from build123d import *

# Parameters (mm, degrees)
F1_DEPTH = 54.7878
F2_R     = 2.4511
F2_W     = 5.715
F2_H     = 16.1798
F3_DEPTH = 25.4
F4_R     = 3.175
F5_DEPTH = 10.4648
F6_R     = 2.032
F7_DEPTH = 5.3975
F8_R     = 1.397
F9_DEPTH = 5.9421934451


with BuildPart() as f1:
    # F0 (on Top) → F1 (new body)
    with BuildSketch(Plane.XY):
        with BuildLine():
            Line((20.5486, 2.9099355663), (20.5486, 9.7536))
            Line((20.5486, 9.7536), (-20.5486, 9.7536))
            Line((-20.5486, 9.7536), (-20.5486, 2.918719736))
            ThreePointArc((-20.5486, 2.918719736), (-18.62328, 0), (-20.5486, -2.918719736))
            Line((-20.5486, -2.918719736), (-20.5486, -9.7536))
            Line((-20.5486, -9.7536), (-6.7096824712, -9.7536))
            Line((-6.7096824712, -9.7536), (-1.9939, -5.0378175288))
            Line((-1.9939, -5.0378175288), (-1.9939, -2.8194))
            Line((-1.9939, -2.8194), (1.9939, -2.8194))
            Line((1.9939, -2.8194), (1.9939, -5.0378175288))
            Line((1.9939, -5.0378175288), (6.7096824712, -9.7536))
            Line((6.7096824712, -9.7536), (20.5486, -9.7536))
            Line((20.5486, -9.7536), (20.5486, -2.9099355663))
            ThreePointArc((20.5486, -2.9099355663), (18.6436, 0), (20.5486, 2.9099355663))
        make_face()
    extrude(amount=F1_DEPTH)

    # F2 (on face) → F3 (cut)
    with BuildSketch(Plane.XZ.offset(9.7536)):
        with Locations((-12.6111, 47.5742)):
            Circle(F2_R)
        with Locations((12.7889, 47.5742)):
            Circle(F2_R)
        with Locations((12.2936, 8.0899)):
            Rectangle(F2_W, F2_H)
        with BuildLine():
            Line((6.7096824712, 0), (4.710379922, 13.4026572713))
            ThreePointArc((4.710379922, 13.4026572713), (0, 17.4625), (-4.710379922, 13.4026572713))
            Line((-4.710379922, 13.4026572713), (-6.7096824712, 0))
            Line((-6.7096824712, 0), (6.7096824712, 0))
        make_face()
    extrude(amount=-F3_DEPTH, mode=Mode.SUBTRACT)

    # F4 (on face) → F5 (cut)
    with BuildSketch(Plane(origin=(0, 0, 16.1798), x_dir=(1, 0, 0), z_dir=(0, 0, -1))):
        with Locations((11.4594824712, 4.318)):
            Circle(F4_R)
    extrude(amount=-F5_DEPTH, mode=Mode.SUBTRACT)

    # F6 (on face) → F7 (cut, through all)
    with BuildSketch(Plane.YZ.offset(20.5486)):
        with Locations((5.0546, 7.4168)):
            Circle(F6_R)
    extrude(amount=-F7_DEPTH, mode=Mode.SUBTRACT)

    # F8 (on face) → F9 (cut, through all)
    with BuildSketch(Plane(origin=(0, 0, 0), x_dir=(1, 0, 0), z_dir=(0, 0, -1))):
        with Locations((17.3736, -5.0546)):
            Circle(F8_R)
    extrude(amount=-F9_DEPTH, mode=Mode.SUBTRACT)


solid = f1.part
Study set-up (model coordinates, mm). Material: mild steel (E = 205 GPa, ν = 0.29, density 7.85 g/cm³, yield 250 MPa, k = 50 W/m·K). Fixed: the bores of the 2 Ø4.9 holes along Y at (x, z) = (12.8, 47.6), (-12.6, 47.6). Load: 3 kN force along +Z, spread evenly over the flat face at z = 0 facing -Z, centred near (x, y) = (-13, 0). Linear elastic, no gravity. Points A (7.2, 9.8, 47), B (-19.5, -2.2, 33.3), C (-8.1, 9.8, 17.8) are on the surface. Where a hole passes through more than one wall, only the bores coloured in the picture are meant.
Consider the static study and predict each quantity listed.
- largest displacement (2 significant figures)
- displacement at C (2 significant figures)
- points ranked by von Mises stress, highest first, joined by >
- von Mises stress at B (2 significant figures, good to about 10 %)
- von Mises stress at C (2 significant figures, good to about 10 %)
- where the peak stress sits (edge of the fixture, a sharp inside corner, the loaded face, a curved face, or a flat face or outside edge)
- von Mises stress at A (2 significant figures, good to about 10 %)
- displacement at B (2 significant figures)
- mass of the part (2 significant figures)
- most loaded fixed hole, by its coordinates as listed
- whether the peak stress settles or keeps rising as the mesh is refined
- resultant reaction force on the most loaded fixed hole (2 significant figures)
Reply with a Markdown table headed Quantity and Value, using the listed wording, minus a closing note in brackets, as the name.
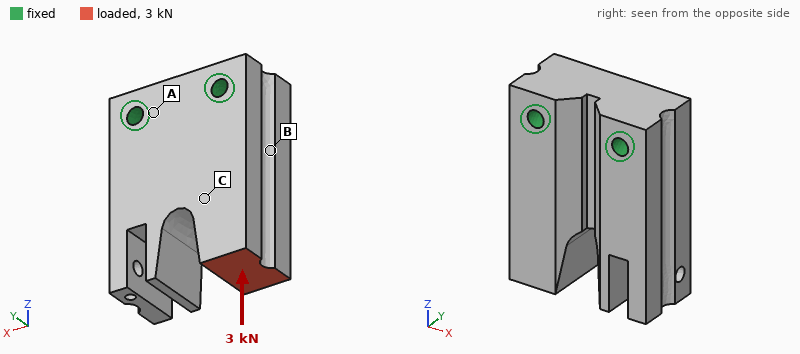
| Quantity | Value |
|---|---|
| largest displacement | 4.4 µm |
| displacement at C | 1.4 µm |
| points ranked by von Mises stress, highest first, joined by > | B > C > A |
| von Mises stress at B | 13 MPa |
| von Mises stress at C | 8.2 MPa |
| where the peak stress sits | edge of the fixture |
| von Mises stress at A | 2.2 MPa |
| displacement at B | 1.0 µm |
| mass of the part | 270 g |
| most loaded fixed hole, by its coordinates as listed | (-12.6, 47.6) |
| whether the peak stress settles or keeps rising as the mesh is refined | keeps rising |
| resultant reaction force on the most loaded fixed hole | 3.0 kN |
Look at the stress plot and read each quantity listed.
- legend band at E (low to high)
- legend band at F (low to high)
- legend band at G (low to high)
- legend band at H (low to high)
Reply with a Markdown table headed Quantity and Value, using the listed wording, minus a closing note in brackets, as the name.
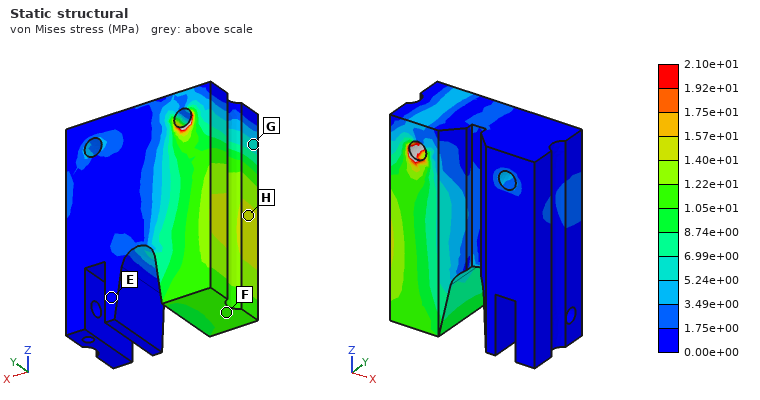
| Quantity | Value |
|---|---|
| legend band at E | 0.00e+00 to 1.75e+00 MPa |
| legend band at F | 1.05e+01 to 1.22e+01 MPa |
| legend band at G | 5.24e+00 to 6.99e+00 MPa |
| legend band at H | 1.40e+01 to 1.57e+01 MPa |
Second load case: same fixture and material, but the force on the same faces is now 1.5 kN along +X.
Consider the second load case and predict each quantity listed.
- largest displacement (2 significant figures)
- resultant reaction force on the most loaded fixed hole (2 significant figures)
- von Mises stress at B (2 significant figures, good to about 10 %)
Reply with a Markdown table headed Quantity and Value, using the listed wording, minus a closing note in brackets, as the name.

| Quantity | Value |
|---|---|
| largest displacement | 13 µm |
| resultant reaction force on the most loaded fixed hole | 2.7 kN |
| von Mises stress at B | 17 MPa |
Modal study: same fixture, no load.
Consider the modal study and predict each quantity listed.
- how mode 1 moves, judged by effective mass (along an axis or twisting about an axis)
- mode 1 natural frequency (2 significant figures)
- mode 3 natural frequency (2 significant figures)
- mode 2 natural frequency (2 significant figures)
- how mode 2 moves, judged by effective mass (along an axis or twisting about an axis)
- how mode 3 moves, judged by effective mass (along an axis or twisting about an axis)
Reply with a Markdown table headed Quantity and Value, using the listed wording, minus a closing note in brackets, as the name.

| Quantity | Value |
|---|---|
| how mode 1 moves, judged by effective mass | along Y |
| mode 1 natural frequency | 7100 Hz |
| mode 3 natural frequency | 11 kHz |
| mode 2 natural frequency | 9300 Hz |
| how mode 2 moves, judged by effective mass | along X |
| how mode 3 moves, judged by effective mass | twisting about Z |
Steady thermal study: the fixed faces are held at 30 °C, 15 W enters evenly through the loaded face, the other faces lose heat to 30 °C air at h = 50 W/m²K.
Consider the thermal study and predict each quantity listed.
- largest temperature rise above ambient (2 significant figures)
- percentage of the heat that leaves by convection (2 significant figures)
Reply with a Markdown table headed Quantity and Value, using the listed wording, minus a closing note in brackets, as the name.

| Quantity | Value |
|---|---|
| largest temperature rise above ambient | 34 K |
| percentage of the heat that leaves by convection | 21 % |
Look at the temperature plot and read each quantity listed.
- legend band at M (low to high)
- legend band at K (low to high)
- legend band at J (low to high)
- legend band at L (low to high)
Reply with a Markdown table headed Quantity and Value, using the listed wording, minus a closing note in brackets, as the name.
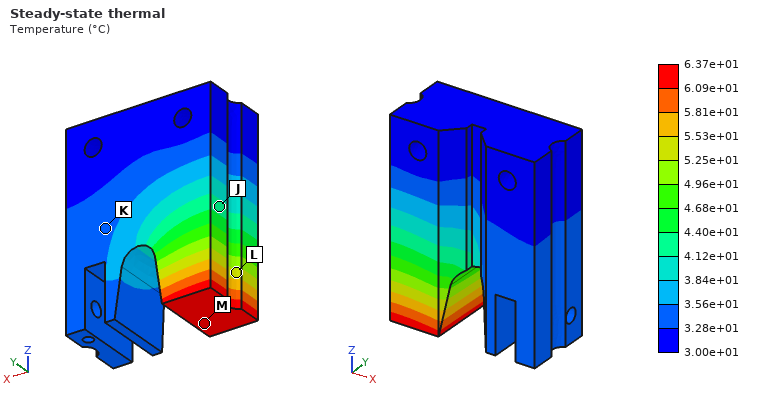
| Quantity | Value |
|---|---|
| legend band at M | 6.09e+01 to 6.37e+01 °C |
| legend band at K | 3.28e+01 to 3.56e+01 °C |
| legend band at J | 4.12e+01 to 4.40e+01 °C |
| legend band at L | 5.25e+01 to 5.53e+01 °C |
